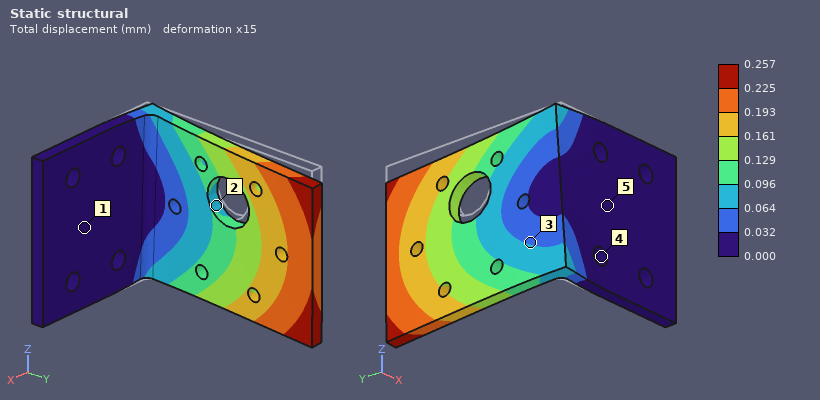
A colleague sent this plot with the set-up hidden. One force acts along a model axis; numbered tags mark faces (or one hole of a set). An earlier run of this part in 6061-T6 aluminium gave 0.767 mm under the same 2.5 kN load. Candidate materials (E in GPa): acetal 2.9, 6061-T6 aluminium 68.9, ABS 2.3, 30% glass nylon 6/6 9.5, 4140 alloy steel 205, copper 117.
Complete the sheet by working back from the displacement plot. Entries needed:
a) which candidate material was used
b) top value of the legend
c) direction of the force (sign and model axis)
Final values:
4140 alloy steel
0.257 mm
-Z
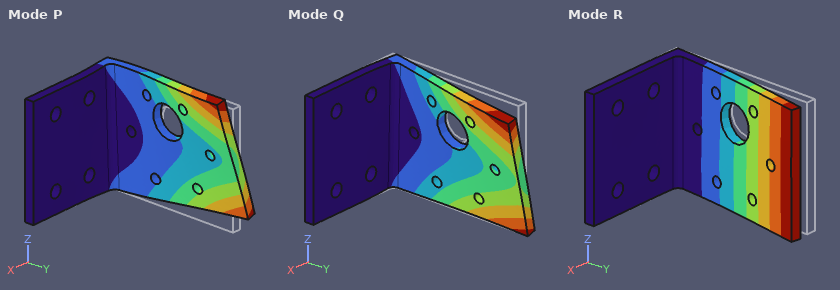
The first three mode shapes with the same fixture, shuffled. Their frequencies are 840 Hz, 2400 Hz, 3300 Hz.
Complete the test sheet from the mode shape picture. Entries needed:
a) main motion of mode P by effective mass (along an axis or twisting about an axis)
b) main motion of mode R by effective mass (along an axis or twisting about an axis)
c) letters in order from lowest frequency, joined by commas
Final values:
along Z
along X
R, Q, P
